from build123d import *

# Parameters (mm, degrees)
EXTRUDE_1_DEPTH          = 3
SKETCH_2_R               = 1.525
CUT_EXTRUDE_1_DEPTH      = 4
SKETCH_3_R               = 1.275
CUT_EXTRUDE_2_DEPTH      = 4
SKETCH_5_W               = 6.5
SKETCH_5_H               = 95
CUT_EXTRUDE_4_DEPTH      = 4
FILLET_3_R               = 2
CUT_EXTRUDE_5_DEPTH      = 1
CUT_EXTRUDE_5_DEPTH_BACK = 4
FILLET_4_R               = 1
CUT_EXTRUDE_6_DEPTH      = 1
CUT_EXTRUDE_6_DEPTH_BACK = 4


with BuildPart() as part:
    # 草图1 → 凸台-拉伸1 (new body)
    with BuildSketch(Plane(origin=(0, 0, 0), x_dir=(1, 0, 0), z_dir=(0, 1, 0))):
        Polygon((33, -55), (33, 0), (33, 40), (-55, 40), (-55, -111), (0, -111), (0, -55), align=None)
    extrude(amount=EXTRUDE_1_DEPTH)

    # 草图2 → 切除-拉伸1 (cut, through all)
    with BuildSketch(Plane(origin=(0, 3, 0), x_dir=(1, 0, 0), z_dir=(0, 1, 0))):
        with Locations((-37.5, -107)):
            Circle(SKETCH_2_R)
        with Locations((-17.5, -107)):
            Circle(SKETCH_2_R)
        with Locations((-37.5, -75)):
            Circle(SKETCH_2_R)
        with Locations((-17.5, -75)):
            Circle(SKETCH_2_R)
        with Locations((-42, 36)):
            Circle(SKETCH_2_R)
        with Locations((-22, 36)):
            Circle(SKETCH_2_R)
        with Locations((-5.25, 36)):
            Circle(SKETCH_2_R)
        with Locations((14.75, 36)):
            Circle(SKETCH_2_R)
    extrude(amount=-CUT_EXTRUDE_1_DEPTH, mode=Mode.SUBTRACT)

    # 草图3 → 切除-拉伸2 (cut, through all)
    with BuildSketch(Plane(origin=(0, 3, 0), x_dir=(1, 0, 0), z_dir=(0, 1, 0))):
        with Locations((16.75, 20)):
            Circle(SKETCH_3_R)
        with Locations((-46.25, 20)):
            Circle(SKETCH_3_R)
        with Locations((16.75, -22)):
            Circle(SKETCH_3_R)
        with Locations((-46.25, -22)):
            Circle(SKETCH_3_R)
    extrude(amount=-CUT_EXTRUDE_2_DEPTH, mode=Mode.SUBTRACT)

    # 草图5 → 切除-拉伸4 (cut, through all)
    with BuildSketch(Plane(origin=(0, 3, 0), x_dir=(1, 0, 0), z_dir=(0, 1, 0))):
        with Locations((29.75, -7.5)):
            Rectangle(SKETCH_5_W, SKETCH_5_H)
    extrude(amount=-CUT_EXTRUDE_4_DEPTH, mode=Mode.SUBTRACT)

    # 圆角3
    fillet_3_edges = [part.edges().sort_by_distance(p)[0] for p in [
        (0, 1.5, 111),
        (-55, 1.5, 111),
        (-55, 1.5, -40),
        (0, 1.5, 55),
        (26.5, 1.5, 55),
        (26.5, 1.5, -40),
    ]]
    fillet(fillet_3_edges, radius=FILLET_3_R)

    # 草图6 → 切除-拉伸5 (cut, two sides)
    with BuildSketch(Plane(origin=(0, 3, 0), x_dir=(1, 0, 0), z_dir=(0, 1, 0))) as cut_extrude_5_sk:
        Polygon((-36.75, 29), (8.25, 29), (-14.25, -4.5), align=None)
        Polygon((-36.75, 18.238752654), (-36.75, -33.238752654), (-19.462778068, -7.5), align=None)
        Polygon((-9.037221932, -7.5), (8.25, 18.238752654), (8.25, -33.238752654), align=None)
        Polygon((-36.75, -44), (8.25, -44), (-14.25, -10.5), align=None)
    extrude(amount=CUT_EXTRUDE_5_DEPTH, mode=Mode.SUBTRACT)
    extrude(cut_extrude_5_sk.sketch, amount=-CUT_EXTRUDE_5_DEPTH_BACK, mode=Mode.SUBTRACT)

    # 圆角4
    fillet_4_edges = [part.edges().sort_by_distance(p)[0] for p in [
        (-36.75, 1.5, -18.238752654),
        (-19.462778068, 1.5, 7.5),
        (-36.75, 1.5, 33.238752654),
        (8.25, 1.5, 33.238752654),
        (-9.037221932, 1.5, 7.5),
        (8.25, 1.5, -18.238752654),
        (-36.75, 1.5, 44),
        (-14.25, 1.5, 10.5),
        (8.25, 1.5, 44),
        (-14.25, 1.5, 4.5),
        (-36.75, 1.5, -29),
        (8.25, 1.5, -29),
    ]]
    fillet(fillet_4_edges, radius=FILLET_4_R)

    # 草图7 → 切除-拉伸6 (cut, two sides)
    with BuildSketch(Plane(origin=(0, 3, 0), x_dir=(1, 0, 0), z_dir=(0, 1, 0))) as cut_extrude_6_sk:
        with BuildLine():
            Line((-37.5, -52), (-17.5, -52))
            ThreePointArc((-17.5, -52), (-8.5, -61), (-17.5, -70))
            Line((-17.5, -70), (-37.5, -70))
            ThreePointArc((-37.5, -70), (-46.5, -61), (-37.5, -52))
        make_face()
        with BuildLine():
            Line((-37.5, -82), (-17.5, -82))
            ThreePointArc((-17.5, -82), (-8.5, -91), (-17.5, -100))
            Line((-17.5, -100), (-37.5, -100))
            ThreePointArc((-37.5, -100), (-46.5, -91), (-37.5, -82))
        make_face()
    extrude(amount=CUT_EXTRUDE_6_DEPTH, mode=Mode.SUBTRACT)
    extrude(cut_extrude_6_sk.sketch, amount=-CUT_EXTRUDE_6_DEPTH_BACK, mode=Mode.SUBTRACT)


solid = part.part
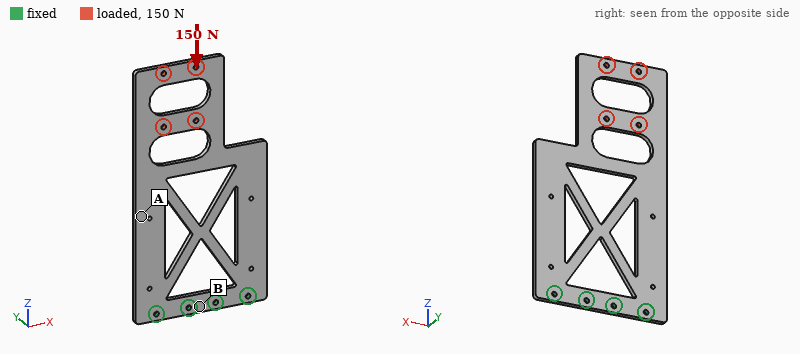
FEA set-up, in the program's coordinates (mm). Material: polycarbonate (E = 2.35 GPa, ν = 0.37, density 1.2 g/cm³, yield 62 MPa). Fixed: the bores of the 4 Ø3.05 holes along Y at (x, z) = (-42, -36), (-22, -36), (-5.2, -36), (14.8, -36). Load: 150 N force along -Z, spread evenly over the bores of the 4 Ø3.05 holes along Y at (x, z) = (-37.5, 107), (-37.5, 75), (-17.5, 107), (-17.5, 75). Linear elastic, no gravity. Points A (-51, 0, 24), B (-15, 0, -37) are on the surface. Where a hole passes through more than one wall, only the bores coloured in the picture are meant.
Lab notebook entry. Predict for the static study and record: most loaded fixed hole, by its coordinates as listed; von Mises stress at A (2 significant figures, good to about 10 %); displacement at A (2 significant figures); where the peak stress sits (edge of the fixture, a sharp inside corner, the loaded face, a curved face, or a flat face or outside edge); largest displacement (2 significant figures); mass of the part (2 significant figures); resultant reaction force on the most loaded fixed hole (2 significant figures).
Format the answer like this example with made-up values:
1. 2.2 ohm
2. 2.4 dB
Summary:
1. (-42, -36)
2. 2.0 MPa
3. 0.090 mm
4. a curved face
5. 0.22 mm
6. 26 g
7. 110 N
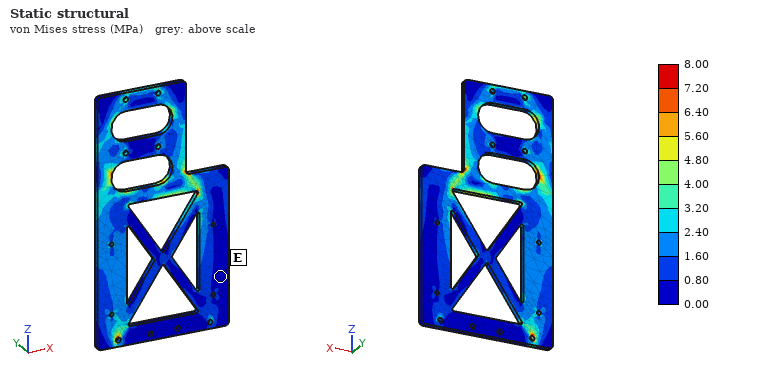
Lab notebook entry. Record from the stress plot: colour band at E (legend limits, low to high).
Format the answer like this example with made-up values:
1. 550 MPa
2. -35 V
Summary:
1. 0.00 to 0.80 MPa
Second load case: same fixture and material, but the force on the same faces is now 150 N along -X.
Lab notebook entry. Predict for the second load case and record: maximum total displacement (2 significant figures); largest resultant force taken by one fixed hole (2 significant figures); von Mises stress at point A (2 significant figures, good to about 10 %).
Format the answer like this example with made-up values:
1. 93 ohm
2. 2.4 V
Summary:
1. 1.7 mm
2. 340 N
3. 5.2 MPa
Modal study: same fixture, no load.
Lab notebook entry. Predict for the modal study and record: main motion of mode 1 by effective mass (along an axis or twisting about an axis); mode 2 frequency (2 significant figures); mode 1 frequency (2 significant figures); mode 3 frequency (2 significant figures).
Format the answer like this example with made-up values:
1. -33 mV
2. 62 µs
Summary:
1. along Y
2. 130 Hz
3. 32 Hz
4. 160 Hz
